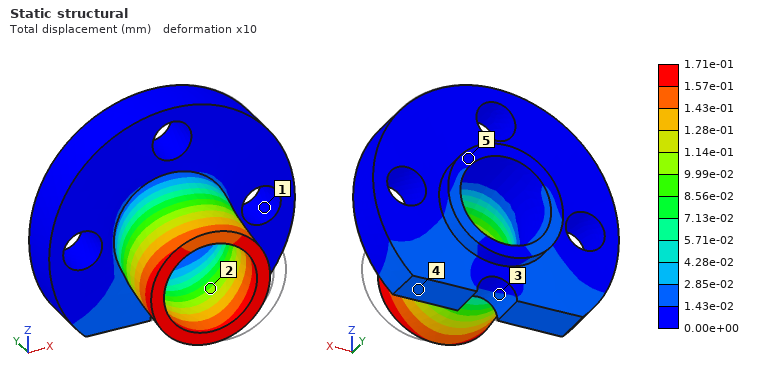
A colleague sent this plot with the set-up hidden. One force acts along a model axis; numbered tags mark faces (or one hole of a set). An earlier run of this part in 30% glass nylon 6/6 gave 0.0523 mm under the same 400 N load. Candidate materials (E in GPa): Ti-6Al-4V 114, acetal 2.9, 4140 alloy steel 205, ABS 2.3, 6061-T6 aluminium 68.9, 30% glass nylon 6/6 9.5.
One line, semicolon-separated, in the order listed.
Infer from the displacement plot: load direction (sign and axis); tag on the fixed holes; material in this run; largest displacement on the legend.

-X; 1; acetal; 1.71e-01 mm
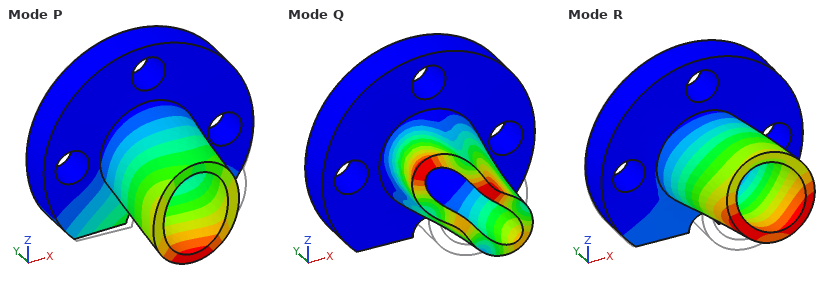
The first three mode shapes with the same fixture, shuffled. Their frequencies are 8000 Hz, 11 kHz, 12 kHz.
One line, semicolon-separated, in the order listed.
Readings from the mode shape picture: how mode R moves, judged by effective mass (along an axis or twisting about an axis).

along X
